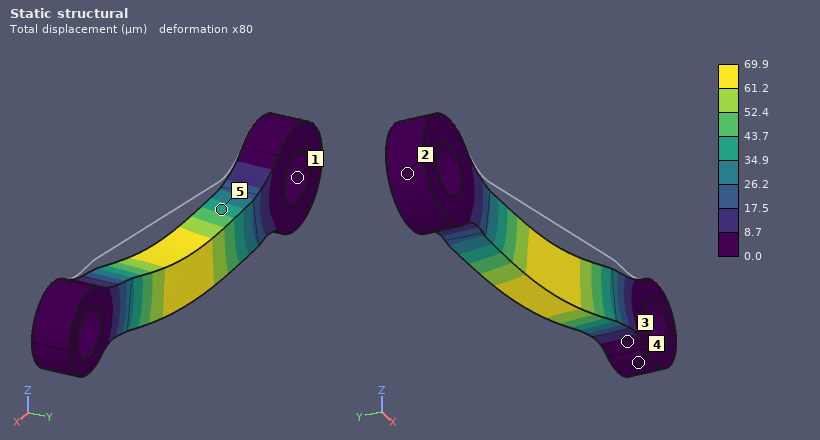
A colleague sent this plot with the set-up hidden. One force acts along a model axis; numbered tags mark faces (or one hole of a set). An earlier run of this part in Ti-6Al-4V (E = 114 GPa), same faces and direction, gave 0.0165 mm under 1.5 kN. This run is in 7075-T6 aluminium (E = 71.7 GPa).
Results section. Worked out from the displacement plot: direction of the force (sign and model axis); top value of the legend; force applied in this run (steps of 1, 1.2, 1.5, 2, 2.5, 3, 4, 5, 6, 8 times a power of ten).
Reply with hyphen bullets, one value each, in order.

- -Z
- 69.9 µm
- 4 kN
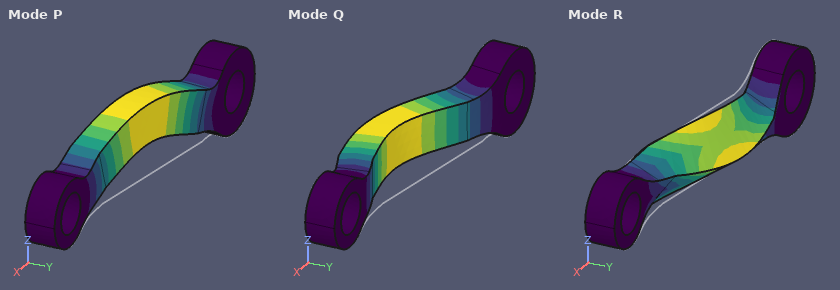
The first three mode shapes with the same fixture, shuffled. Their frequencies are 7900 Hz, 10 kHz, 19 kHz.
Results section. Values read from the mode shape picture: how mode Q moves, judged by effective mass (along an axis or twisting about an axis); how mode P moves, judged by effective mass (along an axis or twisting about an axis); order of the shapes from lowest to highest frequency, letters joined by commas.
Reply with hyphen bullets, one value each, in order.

- along Y
- along Z
- Q, P, R
